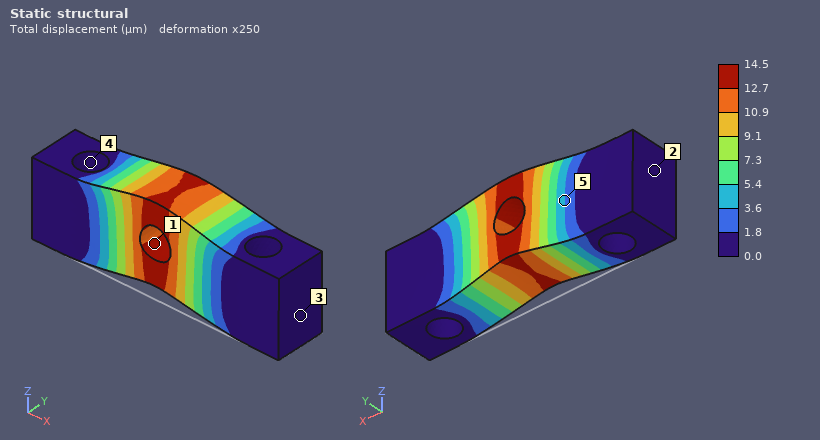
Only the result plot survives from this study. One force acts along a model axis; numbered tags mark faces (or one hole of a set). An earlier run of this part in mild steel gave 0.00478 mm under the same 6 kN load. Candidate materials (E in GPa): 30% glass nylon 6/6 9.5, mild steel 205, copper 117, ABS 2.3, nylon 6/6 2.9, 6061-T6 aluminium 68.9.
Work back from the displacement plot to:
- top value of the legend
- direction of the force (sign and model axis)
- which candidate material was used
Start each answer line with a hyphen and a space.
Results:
- 14.5 µm
- +Z
- 6061-T6 aluminium
